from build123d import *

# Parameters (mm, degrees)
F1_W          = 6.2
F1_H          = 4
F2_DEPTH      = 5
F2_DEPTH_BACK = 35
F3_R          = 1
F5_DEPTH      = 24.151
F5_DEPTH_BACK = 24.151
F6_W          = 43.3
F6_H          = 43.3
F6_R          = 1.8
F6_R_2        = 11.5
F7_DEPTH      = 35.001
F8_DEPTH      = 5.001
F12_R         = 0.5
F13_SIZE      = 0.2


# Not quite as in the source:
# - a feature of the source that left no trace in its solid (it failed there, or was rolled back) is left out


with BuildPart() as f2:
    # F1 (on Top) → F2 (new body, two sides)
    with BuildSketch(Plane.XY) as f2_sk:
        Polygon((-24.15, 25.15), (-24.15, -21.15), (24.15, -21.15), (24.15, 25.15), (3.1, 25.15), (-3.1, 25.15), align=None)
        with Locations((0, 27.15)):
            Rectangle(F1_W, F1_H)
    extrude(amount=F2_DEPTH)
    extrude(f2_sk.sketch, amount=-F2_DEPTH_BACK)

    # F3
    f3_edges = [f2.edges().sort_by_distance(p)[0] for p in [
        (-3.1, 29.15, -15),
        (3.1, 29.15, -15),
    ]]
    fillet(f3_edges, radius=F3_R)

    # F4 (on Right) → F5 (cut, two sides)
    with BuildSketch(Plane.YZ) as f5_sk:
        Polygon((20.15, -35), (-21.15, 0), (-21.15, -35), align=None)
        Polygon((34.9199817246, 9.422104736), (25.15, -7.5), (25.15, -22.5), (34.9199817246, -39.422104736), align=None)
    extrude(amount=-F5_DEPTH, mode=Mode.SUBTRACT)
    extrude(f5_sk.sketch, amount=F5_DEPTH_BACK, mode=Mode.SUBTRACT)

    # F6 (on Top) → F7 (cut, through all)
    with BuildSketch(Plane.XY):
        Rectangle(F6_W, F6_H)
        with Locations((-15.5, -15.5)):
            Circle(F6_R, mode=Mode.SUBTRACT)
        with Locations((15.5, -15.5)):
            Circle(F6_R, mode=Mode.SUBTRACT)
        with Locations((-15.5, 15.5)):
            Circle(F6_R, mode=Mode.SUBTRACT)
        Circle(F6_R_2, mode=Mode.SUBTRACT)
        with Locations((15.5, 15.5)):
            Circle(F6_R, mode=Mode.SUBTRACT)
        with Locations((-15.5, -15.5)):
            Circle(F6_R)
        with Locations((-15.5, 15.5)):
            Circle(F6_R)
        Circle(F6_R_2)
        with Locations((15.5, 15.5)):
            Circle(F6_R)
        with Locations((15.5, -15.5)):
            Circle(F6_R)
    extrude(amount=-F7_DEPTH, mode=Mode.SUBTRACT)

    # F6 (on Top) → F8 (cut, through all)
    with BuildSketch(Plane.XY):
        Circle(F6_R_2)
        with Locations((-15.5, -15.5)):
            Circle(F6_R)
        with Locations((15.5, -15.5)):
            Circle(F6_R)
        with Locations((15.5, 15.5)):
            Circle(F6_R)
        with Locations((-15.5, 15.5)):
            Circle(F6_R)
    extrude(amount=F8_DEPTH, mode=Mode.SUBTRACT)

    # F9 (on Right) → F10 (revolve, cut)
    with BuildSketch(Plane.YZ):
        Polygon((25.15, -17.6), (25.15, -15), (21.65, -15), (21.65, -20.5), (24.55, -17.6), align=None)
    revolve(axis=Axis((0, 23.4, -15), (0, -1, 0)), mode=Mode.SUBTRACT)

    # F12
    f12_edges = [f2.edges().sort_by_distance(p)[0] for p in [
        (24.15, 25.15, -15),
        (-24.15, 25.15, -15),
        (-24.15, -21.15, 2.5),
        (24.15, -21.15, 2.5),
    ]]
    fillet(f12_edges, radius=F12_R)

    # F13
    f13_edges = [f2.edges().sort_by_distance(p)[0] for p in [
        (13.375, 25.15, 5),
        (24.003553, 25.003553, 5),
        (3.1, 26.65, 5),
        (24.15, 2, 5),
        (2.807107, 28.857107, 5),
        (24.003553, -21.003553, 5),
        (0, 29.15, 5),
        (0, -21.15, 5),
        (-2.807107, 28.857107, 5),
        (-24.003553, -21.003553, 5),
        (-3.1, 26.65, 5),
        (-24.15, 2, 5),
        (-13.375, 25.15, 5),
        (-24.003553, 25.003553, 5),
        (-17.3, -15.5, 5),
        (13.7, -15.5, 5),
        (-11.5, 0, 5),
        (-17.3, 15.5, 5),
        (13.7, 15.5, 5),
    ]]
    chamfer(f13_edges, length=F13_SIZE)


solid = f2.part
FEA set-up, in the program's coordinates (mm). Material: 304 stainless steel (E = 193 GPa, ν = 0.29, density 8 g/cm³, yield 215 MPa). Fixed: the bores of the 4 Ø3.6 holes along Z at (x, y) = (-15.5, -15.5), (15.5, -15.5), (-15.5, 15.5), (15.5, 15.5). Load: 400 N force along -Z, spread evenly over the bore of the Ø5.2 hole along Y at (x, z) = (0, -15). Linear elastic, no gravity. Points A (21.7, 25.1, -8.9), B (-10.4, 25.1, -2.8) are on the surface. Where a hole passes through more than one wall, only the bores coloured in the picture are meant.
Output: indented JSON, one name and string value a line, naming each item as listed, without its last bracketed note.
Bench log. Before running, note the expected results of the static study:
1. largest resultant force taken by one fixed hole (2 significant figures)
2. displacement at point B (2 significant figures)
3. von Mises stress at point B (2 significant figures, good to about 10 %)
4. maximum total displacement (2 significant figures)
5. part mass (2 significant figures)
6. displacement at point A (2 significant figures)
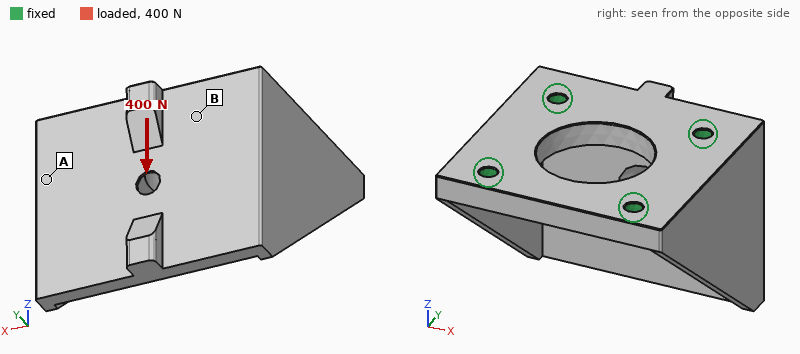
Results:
{
  "largest resultant force taken by one fixed hole": "240 N",
  "displacement at point B": "1.2 µm",
  "von Mises stress at point B": "4.6 MPa",
  "maximum total displacement": "3.9 µm",
  "part mass": "150 g",
  "displacement at point A": "1.0 µm"
}
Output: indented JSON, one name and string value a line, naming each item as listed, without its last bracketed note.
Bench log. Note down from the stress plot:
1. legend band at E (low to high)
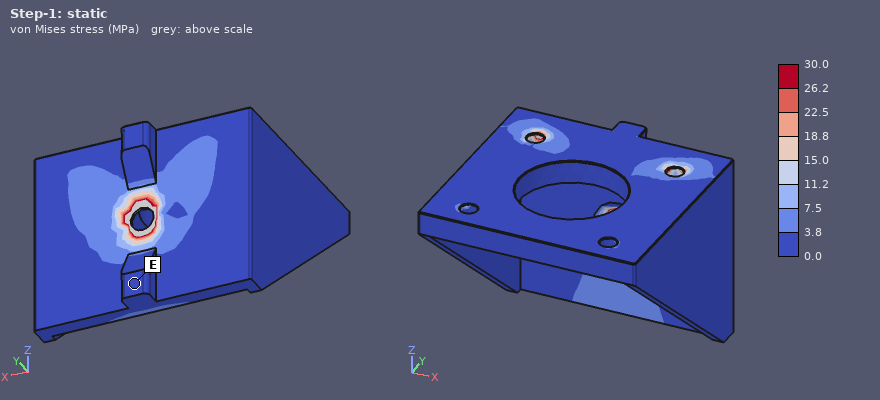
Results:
{
  "legend band at E": "0.0 to 3.8 MPa"
}
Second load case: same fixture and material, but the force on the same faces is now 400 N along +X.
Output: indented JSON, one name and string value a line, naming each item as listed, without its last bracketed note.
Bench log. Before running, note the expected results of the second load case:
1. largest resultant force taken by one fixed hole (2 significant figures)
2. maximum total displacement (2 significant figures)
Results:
{
  "largest resultant force taken by one fixed hole": "300 N",
  "maximum total displacement": "3.0 µm"
}
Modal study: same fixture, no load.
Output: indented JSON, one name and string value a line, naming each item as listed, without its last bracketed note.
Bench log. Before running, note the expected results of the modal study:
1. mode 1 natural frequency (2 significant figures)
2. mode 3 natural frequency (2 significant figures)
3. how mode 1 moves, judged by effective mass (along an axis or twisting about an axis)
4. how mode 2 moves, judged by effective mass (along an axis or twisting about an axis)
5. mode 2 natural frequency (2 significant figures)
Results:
{
  "mode 1 natural frequency": "4700 Hz",
  "mode 3 natural frequency": "8700 Hz",
  "how mode 1 moves, judged by effective mass": "along Y",
  "how mode 2 moves, judged by effective mass": "along X",
  "mode 2 natural frequency": "6800 Hz"
}
